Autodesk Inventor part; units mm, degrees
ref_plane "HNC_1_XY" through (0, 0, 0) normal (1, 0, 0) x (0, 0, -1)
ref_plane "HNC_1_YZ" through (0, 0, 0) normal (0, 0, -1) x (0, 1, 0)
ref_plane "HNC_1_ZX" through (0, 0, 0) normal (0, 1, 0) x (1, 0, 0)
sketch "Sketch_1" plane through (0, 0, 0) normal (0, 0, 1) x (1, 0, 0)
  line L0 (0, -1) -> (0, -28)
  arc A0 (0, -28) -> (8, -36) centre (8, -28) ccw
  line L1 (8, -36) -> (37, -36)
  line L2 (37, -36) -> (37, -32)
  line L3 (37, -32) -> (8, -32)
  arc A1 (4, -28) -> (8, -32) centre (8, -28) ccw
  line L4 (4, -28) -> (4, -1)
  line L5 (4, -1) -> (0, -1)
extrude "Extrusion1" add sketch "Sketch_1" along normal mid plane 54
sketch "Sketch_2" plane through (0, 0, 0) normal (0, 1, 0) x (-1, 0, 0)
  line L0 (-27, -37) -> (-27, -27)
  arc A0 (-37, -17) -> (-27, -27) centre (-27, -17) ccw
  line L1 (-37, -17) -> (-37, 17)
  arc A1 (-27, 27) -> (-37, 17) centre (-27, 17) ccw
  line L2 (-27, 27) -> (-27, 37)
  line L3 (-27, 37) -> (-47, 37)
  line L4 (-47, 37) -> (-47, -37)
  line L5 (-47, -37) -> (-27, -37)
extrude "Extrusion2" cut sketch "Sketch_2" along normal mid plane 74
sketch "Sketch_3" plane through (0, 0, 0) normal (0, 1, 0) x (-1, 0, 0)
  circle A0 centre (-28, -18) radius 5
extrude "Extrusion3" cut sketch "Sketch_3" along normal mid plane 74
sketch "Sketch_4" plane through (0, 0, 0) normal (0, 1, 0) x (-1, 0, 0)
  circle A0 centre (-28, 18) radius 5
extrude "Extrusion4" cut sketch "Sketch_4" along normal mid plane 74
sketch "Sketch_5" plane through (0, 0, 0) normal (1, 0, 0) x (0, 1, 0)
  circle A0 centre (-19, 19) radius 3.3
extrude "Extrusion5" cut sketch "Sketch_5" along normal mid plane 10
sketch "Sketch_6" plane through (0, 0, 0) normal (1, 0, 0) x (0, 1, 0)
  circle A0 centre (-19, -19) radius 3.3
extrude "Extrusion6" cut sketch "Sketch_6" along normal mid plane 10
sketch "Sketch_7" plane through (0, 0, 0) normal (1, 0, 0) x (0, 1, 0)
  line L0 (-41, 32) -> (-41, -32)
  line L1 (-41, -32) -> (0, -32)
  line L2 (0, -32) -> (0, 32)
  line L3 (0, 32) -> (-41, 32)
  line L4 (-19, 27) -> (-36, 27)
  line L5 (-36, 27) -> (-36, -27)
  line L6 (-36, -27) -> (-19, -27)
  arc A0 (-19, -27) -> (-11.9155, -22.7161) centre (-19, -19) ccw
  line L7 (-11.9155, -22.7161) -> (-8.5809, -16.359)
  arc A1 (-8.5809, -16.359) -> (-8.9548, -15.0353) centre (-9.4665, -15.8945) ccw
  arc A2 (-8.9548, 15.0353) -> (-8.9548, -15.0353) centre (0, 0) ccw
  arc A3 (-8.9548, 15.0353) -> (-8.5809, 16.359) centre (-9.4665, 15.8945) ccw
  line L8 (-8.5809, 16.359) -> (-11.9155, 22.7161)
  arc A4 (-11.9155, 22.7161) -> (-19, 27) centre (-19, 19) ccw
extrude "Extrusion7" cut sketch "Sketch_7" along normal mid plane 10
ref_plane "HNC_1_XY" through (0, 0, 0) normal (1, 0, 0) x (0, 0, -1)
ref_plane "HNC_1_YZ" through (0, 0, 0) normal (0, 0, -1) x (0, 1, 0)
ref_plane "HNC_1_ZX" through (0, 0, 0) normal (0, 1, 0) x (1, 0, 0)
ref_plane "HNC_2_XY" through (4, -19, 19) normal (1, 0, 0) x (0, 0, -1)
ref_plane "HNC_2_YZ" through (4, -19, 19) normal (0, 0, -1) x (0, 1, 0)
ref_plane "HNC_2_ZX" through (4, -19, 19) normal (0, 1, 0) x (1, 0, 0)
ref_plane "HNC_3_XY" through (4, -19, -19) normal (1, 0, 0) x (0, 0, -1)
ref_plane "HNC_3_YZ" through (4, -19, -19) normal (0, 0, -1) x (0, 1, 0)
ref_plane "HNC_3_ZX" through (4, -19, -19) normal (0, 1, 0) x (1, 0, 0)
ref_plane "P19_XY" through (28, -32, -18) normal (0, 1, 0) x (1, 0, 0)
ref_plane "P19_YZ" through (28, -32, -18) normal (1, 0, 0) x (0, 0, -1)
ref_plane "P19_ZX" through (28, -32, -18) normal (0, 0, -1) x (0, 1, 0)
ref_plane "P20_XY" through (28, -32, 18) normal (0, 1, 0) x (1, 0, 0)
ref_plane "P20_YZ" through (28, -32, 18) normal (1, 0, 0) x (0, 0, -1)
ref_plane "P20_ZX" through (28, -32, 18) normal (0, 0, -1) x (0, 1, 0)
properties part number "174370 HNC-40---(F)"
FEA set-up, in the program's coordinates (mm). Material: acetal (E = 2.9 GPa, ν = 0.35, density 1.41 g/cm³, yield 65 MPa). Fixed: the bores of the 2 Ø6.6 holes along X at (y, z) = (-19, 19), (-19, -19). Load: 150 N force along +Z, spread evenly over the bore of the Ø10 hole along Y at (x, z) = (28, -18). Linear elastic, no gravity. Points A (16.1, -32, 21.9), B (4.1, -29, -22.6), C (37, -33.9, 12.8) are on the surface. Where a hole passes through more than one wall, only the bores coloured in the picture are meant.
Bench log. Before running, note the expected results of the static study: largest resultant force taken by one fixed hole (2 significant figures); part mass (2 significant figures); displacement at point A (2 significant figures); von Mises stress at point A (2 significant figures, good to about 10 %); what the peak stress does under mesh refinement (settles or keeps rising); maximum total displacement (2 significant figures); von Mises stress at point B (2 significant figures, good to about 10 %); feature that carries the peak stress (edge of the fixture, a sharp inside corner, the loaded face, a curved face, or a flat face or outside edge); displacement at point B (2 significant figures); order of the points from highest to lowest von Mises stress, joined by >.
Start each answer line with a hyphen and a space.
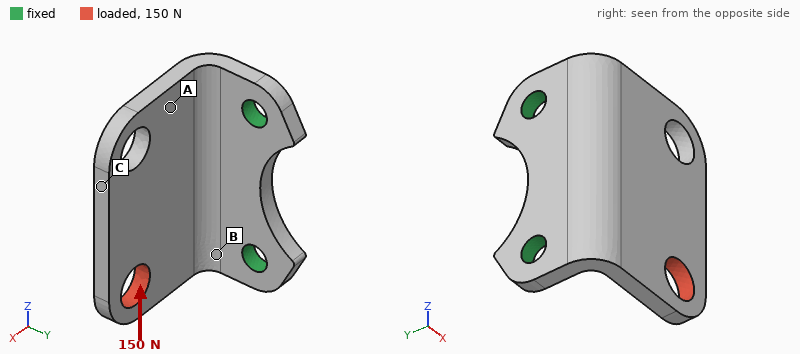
- 130 N
- 15 g
- 0.24 mm
- 3.6 MPa
- keeps rising
- 0.43 mm
- 6.3 MPa
- edge of the fixture
- 0.099 mm
- B > A > C
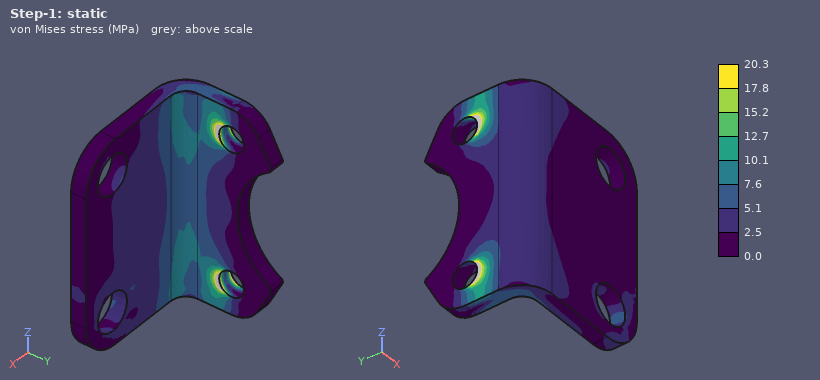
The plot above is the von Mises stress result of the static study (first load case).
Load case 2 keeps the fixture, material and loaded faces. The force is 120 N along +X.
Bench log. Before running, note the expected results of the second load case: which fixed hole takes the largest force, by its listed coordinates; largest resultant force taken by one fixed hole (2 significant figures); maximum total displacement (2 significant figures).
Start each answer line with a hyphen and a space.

- (-19, -19)
- 110 N
- 0.72 mm
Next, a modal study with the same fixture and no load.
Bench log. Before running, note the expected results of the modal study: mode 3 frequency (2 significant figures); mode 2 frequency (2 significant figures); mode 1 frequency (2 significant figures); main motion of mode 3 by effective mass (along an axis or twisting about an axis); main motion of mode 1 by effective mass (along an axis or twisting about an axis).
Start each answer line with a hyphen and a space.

- 1900 Hz
- 1100 Hz
- 540 Hz
- along Z
- along Y
